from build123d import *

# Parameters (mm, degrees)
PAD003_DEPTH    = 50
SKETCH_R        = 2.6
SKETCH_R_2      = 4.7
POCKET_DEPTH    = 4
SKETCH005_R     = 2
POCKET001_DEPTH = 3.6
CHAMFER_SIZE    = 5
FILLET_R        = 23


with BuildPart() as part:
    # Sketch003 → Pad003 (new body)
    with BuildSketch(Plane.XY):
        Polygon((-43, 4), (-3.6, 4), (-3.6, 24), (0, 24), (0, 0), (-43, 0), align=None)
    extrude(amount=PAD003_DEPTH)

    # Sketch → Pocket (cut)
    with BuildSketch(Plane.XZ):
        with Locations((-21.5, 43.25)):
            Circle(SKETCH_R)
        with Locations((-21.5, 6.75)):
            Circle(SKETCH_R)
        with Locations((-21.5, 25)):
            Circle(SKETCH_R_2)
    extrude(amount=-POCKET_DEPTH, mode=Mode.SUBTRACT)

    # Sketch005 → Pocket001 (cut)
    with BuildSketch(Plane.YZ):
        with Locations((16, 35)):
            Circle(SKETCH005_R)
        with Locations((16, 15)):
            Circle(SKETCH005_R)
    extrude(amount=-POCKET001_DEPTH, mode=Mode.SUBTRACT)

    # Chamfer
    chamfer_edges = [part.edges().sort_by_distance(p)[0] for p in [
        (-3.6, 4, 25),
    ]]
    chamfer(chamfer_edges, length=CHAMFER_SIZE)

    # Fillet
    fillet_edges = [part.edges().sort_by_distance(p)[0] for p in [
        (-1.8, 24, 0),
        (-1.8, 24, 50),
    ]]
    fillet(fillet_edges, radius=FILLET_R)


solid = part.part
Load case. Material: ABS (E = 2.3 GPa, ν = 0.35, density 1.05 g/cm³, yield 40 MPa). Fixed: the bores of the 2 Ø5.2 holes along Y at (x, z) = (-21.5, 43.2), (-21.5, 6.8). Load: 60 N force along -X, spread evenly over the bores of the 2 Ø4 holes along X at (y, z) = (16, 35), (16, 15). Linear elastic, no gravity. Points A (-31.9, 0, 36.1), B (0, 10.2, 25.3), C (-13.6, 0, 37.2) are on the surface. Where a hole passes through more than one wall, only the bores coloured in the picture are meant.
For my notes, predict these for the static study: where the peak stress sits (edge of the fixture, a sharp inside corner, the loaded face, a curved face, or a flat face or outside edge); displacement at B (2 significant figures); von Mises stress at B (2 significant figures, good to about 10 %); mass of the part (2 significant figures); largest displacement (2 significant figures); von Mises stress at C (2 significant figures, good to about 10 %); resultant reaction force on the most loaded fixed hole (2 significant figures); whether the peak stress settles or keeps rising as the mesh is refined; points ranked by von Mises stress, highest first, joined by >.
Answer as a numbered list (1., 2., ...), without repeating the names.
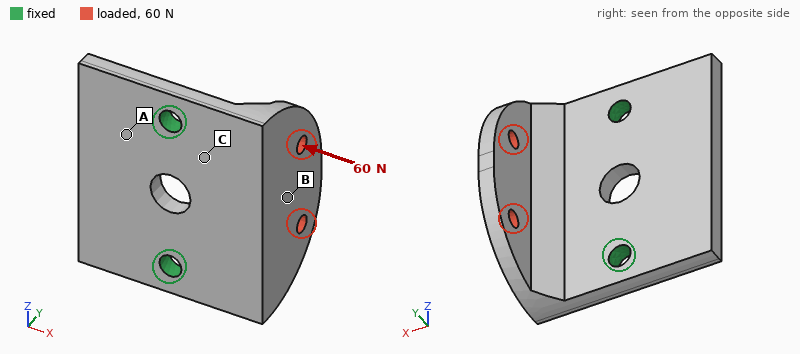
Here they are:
1. edge of the fixture
2. 0.35 mm
3. 3.2 MPa
4. 12 g
5. 0.63 mm
6. 5.3 MPa
7. 31 N
8. keeps rising
9. C > B > A
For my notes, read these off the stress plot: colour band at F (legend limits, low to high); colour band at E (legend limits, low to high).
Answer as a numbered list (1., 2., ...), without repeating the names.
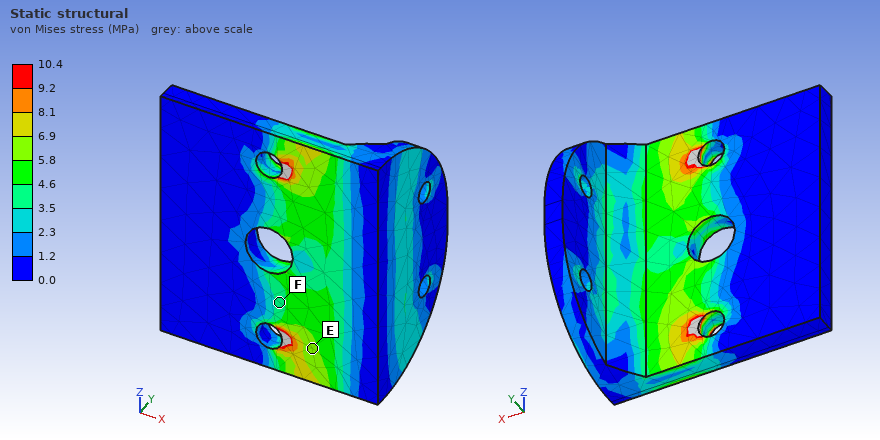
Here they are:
1. 3.5 to 4.6 MPa
2. 5.8 to 6.9 MPa
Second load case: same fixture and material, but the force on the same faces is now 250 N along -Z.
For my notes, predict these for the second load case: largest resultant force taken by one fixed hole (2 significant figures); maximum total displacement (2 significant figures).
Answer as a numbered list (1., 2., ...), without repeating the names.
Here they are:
1. 200 N
2. 0.43 mm
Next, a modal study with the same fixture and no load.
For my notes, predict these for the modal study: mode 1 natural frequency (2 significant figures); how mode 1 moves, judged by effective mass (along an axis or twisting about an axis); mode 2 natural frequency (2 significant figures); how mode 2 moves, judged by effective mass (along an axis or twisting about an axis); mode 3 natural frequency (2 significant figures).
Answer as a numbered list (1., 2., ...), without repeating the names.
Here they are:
1. 920 Hz
2. along Y
3. 1900 Hz
4. along Y
5. 2000 Hz
